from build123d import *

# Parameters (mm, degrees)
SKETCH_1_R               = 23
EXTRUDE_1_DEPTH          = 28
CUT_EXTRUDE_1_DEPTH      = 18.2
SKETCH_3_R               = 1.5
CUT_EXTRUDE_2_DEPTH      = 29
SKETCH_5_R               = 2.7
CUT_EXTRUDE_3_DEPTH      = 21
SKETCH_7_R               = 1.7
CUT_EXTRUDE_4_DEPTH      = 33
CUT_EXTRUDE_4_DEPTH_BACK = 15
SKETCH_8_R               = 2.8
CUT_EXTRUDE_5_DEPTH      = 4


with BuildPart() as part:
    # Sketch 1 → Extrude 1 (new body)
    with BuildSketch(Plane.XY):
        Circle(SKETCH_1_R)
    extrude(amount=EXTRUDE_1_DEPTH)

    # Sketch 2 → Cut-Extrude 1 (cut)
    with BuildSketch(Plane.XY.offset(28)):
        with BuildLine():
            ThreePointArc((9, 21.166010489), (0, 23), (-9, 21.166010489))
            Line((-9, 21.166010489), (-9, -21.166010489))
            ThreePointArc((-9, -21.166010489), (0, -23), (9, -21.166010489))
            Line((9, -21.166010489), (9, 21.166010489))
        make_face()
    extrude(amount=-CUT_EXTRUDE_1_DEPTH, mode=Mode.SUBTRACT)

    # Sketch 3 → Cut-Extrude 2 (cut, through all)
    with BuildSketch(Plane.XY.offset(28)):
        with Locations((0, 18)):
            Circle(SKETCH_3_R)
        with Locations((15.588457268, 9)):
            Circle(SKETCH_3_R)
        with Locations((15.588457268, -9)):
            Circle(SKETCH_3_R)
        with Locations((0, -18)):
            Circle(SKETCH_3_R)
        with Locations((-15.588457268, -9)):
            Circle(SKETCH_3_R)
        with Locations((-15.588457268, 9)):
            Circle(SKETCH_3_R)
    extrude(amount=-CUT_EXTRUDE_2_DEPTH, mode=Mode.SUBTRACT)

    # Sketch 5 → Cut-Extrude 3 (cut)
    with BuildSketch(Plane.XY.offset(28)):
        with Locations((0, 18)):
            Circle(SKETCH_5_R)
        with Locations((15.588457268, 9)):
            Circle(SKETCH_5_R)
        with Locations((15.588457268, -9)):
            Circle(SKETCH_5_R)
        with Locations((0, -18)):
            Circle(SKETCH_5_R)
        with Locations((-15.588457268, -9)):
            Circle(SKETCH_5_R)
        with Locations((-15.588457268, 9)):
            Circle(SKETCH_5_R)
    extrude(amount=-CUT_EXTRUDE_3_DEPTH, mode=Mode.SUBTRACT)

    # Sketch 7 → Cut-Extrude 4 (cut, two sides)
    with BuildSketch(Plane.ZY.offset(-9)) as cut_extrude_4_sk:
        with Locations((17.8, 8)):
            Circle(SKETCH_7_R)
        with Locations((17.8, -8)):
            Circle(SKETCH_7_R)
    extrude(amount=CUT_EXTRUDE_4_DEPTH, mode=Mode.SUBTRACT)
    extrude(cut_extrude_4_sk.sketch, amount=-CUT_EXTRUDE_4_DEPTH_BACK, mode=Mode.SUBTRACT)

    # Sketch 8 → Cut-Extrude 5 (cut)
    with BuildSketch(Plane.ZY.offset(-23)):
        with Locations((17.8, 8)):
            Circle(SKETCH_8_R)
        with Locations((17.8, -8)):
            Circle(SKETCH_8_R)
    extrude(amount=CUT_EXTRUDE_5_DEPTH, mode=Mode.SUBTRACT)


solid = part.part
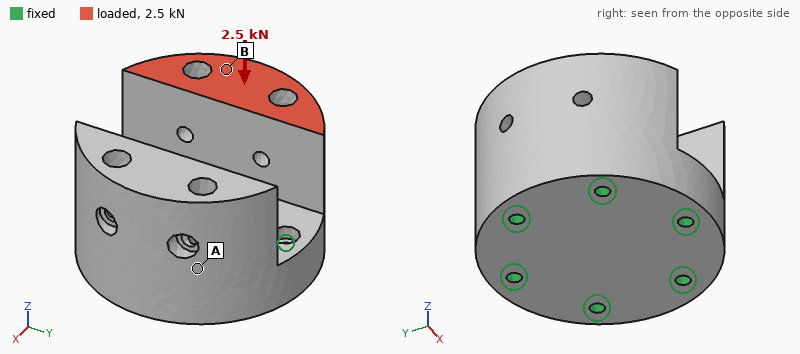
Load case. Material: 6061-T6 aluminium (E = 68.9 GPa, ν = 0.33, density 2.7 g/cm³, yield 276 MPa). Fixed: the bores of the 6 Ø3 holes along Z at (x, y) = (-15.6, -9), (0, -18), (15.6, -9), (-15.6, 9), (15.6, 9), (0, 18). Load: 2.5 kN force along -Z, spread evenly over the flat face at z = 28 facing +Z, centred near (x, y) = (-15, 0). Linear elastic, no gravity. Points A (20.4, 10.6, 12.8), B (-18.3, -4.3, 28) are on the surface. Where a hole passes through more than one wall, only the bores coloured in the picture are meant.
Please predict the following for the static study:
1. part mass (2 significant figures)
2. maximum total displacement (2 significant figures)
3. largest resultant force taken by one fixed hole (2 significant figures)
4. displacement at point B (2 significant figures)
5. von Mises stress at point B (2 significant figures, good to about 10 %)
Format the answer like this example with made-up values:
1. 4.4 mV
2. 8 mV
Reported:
1. 79 g
2. 4.7 µm
3. 1.1 kN
4. 4.4 µm
5. 6.7 MPa
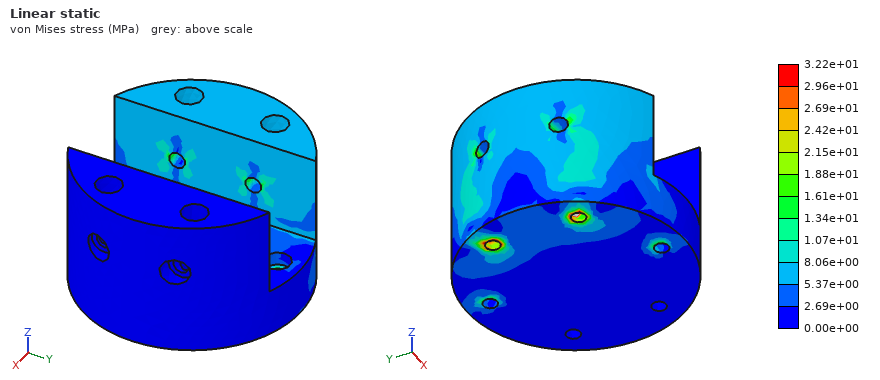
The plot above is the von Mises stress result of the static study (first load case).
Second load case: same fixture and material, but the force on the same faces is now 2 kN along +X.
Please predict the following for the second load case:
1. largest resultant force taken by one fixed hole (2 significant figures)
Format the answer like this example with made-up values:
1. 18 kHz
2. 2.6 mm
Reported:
1. 1.1 kN
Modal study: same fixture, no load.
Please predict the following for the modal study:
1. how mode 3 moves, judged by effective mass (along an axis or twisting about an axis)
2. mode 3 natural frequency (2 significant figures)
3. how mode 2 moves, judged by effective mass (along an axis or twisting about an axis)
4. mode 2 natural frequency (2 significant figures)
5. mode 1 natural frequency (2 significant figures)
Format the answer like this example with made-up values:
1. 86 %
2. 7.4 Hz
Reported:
1. along Y
2. 19 kHz
3. along X
4. 13 kHz
5. 13 kHz
